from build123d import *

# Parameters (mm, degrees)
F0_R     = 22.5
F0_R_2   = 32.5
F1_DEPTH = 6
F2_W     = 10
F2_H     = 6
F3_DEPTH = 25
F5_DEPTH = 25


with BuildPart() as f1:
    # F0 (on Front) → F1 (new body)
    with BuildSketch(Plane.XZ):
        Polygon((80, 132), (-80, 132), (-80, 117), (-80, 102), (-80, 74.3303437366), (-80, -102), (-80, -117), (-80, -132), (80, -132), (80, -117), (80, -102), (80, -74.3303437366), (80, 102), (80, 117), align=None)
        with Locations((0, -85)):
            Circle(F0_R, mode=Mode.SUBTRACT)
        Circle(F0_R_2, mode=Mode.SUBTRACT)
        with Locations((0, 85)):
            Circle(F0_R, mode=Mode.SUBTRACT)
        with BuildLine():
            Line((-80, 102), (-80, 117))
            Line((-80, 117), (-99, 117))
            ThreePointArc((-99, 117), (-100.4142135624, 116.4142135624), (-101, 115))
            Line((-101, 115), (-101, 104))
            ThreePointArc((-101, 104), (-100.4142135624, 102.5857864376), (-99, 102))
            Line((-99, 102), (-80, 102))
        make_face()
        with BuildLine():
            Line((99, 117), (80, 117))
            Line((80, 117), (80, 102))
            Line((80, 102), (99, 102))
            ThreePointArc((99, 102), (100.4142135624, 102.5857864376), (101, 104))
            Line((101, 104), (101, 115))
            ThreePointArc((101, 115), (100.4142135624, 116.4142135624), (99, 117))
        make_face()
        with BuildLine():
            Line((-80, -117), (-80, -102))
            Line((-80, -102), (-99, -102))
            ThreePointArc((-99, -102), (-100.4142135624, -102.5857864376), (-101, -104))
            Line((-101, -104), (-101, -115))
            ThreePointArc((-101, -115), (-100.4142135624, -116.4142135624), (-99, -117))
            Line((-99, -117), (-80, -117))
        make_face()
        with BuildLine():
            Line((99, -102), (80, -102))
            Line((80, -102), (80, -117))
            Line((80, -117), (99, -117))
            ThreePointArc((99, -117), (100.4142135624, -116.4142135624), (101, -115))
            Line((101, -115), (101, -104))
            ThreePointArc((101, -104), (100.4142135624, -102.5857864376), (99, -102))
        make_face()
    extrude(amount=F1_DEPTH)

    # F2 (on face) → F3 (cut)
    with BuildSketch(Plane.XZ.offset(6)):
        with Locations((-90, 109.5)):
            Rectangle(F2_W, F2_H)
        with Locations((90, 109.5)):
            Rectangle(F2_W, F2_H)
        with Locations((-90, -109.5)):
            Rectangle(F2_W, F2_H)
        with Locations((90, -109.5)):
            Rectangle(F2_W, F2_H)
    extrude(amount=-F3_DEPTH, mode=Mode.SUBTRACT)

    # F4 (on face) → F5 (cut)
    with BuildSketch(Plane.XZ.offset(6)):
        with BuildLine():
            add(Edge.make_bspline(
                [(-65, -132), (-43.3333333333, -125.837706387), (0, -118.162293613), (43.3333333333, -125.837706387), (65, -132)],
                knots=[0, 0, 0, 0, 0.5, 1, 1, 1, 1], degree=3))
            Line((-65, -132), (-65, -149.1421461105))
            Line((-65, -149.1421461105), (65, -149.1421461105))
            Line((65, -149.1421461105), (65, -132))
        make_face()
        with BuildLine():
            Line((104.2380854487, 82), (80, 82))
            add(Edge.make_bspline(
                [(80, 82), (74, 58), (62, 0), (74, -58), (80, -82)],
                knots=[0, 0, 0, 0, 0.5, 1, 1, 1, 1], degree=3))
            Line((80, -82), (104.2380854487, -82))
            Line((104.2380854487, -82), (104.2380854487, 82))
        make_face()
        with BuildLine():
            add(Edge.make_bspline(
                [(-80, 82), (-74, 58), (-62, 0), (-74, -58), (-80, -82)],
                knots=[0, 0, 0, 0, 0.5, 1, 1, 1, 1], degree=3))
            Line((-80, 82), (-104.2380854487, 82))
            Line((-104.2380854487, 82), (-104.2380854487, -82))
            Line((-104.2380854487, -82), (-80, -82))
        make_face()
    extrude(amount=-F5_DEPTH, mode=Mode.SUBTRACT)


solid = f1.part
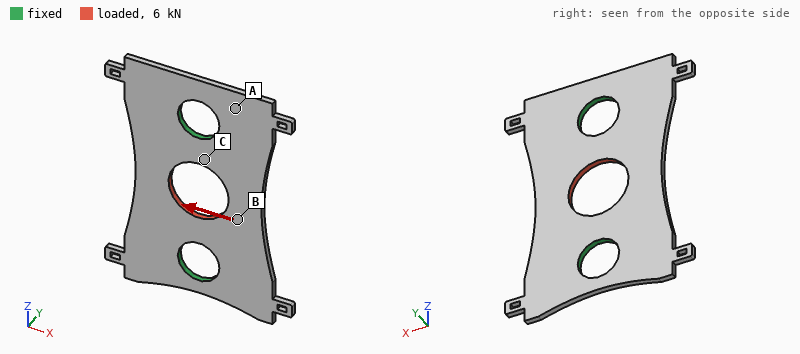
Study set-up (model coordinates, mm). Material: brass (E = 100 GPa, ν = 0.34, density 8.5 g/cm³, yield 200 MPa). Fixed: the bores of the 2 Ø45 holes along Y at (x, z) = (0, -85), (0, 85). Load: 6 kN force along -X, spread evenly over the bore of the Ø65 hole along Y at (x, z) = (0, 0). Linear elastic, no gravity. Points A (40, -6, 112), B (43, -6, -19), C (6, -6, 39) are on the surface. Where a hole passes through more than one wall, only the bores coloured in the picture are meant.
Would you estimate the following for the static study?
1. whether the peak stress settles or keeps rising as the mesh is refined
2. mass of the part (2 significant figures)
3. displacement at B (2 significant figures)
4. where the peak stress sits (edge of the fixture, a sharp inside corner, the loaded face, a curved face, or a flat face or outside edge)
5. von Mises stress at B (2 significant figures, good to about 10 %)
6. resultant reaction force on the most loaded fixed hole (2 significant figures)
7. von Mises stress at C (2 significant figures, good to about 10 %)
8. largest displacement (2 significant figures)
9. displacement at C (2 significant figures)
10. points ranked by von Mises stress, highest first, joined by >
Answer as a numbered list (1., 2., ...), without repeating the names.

1. keeps rising
2. 1.7 kg
3. 7.3 µm
4. edge of the fixture
5. 6.4 MPa
6. 3.0 kN
7. 9.5 MPa
8. 9.0 µm
9. 4.8 µm
10. C > B > A
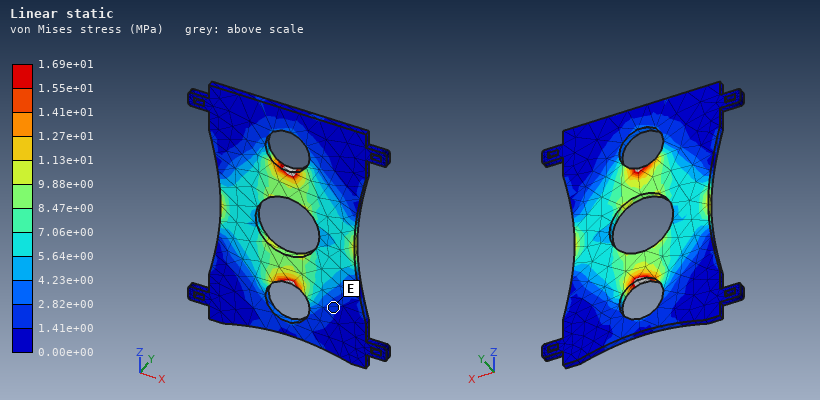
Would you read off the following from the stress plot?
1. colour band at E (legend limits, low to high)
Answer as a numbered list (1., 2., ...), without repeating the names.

1. 1.41e+00 to 2.82e+00 MPa
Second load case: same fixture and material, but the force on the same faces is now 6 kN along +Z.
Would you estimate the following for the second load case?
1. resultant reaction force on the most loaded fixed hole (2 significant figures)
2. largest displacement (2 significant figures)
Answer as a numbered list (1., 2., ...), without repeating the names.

1. 3.0 kN
2. 4.3 µm
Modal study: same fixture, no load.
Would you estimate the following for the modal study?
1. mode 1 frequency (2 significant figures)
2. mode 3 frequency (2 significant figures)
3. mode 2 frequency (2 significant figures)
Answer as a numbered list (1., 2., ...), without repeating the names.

1. 730 Hz
2. 810 Hz
3. 740 Hz
